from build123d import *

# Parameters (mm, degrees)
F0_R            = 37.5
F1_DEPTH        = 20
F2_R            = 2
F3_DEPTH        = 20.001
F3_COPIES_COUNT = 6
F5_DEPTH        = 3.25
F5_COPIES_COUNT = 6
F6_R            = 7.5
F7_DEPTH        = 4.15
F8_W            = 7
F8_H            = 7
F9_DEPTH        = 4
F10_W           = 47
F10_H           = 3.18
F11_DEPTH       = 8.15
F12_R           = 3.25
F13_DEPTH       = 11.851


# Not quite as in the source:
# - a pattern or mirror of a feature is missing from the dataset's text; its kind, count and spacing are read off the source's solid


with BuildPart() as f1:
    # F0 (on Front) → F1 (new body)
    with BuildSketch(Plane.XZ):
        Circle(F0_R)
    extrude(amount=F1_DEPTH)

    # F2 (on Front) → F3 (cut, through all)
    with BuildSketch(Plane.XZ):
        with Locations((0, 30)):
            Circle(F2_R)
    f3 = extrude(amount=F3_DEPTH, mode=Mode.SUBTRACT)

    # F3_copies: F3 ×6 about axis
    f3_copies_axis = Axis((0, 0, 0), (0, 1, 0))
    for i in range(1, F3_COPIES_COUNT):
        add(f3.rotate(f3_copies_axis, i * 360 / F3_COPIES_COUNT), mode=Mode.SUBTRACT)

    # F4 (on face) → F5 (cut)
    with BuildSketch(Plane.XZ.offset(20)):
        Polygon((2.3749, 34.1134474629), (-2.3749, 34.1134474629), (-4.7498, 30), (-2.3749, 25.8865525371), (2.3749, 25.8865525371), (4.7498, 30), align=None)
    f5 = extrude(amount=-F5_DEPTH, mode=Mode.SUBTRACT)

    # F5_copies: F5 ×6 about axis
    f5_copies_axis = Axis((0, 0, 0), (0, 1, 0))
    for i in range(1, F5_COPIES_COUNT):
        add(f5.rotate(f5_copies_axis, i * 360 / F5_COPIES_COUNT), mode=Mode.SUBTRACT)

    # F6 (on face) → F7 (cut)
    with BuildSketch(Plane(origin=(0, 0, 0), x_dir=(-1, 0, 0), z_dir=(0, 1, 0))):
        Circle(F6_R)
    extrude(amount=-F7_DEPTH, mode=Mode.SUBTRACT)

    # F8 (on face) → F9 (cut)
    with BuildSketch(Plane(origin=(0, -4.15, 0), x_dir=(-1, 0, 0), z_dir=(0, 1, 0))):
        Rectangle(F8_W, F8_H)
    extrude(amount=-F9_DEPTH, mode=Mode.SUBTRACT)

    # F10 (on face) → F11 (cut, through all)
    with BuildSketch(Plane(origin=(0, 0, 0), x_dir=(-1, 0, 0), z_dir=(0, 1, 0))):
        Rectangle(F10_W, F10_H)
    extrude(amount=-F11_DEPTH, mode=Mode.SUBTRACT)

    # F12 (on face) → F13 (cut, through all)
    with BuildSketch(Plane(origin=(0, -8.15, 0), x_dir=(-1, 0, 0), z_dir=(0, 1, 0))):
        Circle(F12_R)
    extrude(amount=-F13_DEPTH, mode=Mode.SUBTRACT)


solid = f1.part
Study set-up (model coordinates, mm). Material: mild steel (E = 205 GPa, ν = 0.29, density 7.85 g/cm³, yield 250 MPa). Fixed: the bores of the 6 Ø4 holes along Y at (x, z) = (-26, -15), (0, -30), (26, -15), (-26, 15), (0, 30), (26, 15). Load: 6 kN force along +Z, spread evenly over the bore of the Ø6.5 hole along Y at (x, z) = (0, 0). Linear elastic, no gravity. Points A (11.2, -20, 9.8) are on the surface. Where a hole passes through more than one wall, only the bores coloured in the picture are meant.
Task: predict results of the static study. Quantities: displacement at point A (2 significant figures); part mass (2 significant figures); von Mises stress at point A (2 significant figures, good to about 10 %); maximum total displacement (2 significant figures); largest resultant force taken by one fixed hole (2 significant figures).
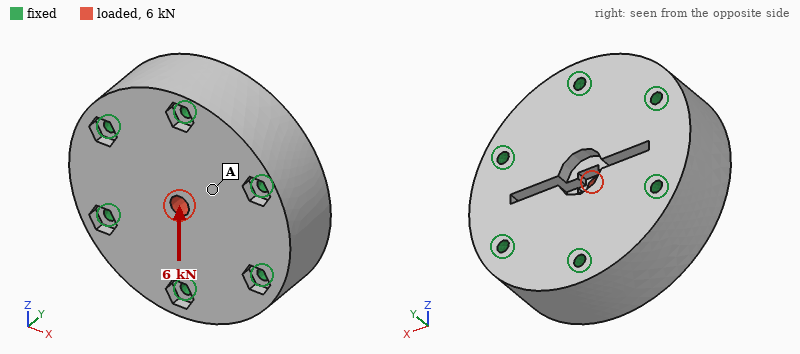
0.50 µm
660 g
5.8 MPa
1.5 µm
1.6 kN
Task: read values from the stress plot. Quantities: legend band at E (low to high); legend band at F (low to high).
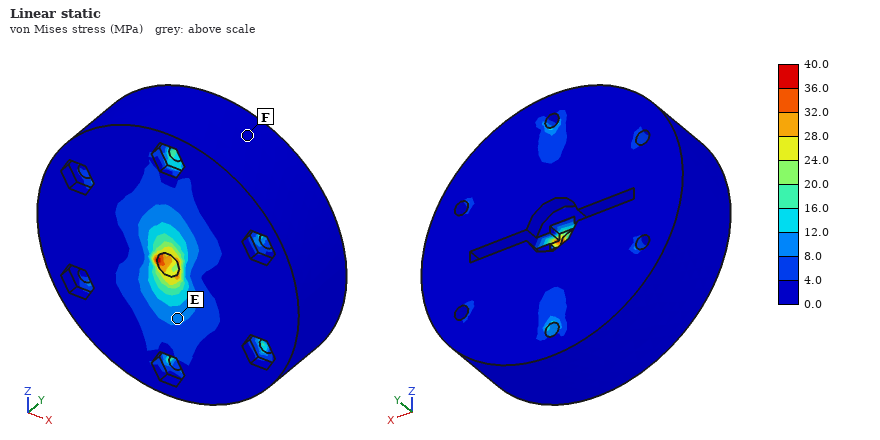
8.0 to 12.0 MPa
0.0 to 4.0 MPa
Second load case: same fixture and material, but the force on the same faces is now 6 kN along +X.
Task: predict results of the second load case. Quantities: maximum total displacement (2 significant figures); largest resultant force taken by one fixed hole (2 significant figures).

1.5 µm
1.4 kN
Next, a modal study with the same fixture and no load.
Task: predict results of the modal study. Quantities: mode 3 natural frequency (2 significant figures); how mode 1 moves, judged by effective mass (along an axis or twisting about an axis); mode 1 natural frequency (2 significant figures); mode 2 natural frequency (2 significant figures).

35 kHz
along Y
23 kHz
34 kHz
